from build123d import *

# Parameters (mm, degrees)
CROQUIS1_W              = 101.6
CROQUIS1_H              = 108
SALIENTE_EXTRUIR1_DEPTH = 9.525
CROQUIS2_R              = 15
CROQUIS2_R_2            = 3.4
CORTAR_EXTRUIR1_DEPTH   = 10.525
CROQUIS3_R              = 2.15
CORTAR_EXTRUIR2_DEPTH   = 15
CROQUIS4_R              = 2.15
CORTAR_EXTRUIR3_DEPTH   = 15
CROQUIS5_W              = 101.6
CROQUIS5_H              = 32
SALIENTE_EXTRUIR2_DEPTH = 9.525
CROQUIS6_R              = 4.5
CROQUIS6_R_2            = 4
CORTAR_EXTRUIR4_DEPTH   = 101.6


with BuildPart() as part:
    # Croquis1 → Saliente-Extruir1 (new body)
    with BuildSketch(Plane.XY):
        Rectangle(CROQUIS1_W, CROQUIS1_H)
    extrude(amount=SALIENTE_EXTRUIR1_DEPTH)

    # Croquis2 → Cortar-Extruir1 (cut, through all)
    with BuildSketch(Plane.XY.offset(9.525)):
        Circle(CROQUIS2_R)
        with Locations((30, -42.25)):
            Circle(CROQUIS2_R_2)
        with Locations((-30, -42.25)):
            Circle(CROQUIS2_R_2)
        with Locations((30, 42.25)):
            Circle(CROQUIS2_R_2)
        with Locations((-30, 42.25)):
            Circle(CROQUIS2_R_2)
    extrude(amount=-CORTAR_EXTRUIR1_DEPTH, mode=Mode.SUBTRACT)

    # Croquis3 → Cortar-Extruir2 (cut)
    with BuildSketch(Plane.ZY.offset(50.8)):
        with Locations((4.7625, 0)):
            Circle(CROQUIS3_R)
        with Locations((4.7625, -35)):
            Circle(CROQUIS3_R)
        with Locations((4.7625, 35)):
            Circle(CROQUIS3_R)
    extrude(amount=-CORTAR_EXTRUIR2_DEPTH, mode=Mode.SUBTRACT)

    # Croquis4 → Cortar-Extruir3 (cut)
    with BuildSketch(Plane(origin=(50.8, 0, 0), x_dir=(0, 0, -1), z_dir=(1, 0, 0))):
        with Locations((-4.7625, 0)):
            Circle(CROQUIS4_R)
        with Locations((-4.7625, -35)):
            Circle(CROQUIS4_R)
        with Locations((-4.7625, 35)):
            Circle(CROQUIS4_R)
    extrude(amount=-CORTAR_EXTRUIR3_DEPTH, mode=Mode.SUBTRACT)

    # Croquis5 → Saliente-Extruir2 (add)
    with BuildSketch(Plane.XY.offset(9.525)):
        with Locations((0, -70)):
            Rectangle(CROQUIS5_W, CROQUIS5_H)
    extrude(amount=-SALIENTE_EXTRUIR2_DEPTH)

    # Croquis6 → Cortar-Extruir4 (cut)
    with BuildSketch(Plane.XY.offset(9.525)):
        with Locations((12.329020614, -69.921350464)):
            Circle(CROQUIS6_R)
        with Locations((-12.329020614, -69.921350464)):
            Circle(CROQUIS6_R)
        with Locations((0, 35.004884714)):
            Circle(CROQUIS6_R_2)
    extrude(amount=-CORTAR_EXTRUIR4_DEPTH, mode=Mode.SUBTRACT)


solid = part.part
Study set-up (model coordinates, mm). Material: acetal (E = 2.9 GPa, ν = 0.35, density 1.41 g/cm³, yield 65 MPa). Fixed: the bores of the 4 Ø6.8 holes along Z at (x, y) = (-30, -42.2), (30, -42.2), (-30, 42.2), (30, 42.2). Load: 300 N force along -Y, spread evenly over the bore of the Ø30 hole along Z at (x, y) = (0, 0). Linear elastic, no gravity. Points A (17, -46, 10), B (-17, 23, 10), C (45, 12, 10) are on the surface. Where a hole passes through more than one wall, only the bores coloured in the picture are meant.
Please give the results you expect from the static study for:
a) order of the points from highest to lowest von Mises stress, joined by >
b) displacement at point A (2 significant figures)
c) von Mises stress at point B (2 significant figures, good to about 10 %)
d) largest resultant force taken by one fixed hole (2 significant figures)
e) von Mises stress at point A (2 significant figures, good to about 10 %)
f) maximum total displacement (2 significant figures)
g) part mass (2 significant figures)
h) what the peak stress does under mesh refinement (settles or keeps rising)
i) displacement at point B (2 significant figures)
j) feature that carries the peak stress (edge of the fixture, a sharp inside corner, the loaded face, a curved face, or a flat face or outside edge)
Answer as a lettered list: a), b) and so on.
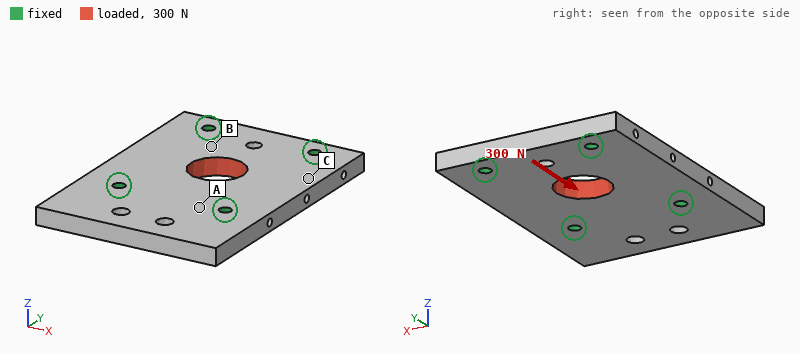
a) B > A > C
b) 1.6 µm
c) 0.31 MPa
d) 80 N
e) 0.16 MPa
f) 5.4 µm
g) 180 g
h) keeps rising
i) 3.1 µm
j) edge of the fixture
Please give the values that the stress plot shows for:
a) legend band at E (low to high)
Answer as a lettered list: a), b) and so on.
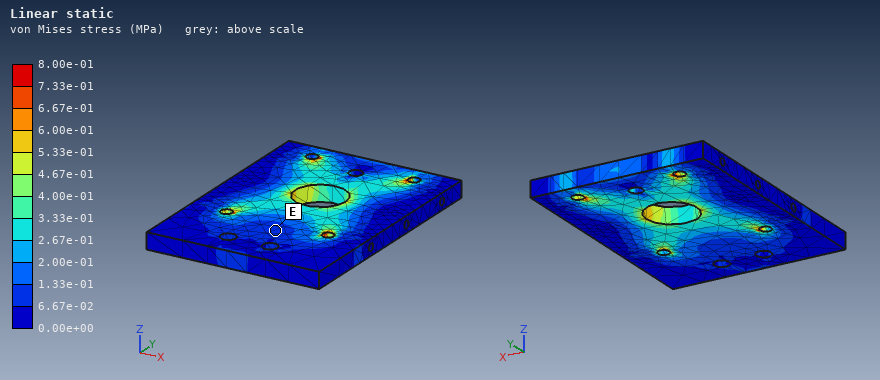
a) 6.67e-02 to 1.33e-01 MPa
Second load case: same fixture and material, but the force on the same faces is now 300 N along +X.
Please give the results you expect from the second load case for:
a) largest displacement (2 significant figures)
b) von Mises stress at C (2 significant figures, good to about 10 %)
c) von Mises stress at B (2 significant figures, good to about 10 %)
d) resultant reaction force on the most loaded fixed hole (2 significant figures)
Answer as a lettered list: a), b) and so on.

a) 8.2 µm
b) 0.19 MPa
c) 0.31 MPa
d) 85 N
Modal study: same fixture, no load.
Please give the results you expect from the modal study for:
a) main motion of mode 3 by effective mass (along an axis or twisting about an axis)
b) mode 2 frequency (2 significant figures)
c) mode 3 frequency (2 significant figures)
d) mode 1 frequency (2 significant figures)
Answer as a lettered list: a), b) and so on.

a) along Z
b) 1400 Hz
c) 1700 Hz
d) 1000 Hz
